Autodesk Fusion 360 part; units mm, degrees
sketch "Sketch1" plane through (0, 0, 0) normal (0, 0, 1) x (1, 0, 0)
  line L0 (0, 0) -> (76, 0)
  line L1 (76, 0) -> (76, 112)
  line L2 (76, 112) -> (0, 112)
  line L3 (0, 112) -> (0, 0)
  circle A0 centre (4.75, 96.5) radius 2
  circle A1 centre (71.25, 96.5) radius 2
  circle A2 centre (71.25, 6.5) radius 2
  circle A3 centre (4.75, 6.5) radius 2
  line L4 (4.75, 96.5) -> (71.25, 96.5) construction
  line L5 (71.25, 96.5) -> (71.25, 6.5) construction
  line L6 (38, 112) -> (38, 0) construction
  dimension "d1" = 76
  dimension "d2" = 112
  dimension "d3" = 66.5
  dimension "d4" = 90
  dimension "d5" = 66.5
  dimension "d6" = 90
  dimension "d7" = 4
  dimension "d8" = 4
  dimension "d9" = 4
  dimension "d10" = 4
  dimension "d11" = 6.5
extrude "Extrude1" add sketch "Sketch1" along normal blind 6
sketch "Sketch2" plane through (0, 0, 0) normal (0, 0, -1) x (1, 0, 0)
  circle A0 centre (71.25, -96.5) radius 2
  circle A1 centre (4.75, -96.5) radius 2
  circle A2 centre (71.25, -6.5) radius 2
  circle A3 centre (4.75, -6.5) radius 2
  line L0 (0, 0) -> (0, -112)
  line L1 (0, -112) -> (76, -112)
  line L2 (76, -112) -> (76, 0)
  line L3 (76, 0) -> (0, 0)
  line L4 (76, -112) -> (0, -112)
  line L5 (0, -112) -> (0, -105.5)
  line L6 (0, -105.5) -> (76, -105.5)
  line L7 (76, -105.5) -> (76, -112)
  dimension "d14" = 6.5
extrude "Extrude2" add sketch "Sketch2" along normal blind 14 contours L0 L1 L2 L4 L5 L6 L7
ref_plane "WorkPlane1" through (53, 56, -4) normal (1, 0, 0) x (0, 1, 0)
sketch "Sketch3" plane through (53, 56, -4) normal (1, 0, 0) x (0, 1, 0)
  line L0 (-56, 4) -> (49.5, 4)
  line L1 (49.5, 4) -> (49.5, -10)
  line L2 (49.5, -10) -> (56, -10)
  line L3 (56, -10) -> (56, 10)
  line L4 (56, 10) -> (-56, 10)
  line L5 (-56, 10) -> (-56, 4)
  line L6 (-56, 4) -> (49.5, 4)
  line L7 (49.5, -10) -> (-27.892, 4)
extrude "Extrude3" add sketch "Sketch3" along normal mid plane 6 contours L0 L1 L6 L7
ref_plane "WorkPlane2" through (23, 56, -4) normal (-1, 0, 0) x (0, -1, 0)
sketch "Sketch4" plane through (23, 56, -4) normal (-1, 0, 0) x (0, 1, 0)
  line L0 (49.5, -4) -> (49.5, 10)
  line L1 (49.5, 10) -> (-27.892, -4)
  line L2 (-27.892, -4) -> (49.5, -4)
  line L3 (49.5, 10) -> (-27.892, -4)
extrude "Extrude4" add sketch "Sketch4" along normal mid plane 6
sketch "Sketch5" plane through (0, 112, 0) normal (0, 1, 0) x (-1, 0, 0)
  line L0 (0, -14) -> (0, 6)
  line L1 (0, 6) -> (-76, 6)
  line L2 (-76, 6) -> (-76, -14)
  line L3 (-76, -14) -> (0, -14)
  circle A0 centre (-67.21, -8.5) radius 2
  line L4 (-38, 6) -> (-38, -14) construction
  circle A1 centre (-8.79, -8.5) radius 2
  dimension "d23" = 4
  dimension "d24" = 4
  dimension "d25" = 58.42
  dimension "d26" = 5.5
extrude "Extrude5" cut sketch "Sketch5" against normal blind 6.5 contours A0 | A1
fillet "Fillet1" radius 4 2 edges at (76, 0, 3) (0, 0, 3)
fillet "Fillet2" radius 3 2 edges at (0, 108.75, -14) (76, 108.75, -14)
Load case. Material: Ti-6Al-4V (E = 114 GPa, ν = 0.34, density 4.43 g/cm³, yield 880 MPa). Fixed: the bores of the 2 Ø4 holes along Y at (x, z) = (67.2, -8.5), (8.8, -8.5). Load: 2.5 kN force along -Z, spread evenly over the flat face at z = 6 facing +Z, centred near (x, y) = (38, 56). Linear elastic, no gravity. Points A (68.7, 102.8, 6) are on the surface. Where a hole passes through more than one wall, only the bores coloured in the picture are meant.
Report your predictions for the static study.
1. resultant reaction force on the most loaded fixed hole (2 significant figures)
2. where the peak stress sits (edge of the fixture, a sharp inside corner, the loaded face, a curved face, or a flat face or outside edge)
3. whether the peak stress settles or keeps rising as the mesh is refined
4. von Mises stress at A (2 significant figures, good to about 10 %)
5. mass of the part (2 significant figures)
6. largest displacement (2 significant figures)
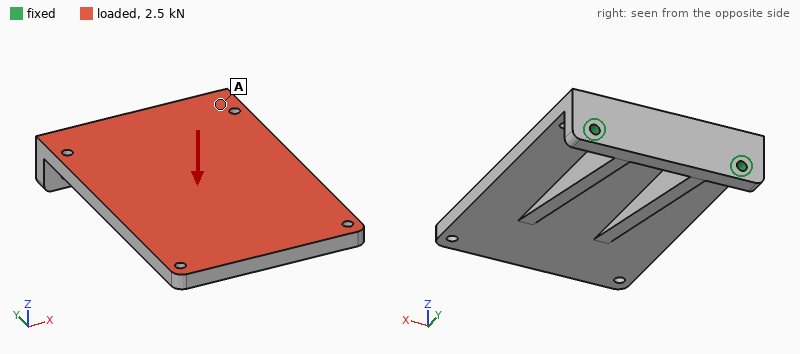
1.6 kN
edge of the fixture
keeps rising
90 MPa
280 g
1.5 mm
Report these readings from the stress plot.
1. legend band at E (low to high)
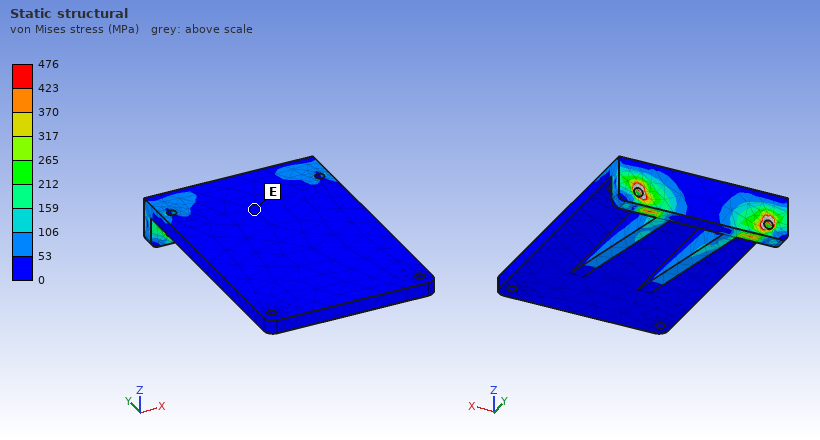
0 to 53 MPa
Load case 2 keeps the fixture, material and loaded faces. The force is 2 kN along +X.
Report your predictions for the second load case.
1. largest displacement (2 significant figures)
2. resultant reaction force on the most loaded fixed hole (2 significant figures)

62 µm
2.1 kN
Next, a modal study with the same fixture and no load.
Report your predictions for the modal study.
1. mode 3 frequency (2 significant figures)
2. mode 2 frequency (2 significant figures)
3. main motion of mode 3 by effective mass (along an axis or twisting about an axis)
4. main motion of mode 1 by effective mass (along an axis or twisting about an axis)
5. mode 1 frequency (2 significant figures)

2300 Hz
1400 Hz
along X
along Z
520 Hz
